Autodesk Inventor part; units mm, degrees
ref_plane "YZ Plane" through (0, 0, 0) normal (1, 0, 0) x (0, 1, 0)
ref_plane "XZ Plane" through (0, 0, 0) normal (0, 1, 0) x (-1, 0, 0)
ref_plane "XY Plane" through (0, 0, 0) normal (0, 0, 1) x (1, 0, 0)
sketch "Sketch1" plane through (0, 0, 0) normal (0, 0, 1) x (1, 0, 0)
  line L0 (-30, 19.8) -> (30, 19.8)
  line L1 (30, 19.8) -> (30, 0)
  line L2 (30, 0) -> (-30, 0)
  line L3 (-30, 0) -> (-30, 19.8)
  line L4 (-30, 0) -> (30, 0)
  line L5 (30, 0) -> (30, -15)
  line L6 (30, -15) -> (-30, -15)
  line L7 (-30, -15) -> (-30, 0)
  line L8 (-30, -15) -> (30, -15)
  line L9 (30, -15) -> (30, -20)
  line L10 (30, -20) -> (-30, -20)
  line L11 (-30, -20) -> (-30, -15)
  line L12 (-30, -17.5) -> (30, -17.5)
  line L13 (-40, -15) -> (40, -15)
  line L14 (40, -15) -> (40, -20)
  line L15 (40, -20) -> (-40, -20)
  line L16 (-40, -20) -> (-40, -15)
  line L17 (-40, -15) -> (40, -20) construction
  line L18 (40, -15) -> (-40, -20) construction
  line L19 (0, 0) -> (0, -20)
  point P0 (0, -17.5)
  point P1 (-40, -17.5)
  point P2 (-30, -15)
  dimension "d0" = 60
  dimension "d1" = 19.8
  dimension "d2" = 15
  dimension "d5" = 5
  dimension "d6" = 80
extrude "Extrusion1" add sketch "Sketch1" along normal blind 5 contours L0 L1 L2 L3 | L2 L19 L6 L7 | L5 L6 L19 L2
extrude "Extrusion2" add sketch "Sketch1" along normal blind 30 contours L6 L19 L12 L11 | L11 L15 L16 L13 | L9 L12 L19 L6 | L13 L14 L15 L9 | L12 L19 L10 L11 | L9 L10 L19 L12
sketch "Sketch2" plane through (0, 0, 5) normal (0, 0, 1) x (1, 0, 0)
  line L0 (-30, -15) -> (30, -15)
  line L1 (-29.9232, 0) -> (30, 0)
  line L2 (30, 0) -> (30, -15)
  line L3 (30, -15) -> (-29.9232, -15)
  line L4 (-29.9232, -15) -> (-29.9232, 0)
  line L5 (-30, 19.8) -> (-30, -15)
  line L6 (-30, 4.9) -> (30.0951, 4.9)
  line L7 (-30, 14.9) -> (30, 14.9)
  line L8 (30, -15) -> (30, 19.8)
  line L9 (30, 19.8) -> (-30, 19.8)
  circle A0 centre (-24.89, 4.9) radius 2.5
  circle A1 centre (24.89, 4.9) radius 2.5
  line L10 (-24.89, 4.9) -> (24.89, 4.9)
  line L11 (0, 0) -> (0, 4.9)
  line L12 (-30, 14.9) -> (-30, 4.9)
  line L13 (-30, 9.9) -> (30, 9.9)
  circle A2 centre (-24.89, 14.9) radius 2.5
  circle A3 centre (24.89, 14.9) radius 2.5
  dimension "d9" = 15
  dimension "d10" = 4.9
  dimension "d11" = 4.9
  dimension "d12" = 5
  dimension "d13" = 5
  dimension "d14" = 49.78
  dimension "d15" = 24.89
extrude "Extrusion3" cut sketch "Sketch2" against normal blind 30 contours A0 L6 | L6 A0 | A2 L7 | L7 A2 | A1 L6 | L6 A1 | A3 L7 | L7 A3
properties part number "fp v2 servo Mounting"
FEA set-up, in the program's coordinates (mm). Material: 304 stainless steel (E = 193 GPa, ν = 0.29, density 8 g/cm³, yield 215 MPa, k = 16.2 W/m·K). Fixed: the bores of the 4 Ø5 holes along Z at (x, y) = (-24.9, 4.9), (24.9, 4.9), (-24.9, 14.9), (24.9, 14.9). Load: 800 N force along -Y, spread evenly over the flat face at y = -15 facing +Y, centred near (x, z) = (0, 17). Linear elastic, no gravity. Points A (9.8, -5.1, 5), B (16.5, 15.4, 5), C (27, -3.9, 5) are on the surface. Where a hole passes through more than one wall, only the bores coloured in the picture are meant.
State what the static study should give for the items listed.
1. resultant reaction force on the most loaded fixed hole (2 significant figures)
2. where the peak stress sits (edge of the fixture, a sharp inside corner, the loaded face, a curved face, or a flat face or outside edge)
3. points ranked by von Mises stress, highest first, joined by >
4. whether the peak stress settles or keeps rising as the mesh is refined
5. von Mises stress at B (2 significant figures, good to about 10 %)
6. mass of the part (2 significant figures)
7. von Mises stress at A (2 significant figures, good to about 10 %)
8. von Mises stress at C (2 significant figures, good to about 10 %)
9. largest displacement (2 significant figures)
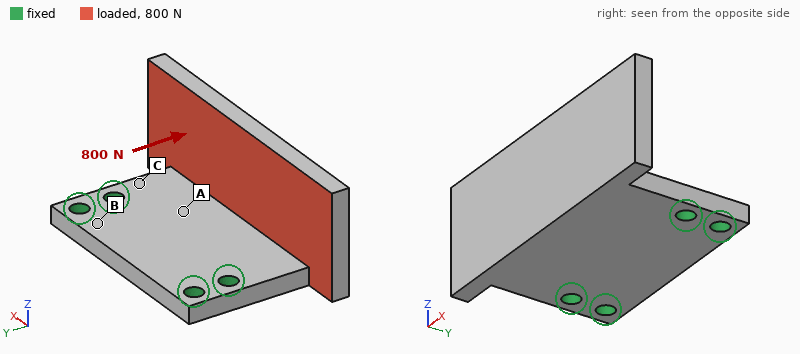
370 N
edge of the fixture
C > A > B
keeps rising
11 MPa
180 g
38 MPa
61 MPa
82 µm
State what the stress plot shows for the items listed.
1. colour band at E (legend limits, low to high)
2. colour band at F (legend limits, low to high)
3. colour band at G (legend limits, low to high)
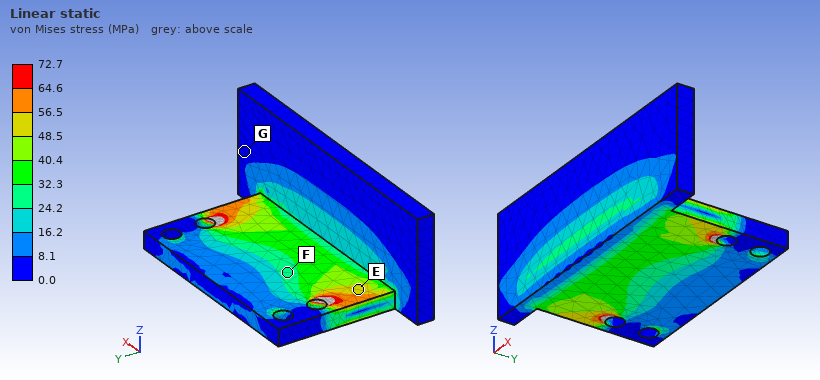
48.5 to 56.5 MPa
24.2 to 32.3 MPa
0.0 to 8.1 MPa
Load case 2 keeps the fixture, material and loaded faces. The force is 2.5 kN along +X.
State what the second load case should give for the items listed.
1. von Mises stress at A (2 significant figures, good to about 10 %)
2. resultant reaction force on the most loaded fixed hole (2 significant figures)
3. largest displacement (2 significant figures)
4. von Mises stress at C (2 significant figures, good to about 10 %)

56 MPa
1.6 kN
78 µm
67 MPa
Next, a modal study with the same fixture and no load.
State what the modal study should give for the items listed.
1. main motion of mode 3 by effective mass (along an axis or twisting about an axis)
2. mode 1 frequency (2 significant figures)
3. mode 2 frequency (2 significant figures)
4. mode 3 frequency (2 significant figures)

along Z
1800 Hz
2800 Hz
4900 Hz
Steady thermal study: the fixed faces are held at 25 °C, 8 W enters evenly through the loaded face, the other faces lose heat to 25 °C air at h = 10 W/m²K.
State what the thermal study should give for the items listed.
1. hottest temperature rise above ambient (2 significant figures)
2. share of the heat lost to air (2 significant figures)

50 K
26 %
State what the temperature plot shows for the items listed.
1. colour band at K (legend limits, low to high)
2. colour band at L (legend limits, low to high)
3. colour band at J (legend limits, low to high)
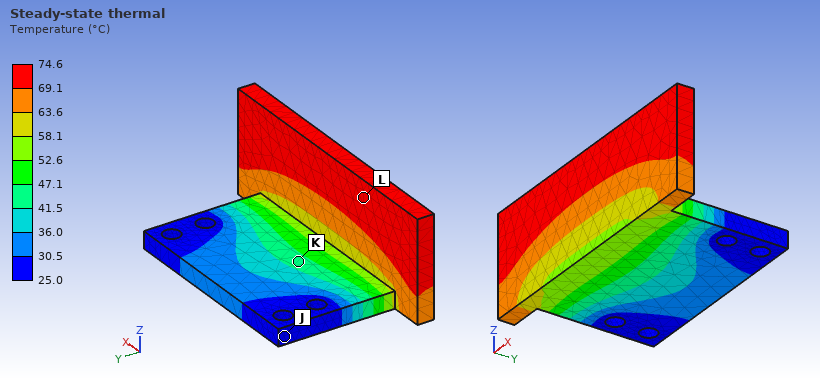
41.5 to 47.1 °C
69.1 to 74.6 °C
25.0 to 30.5 °C
